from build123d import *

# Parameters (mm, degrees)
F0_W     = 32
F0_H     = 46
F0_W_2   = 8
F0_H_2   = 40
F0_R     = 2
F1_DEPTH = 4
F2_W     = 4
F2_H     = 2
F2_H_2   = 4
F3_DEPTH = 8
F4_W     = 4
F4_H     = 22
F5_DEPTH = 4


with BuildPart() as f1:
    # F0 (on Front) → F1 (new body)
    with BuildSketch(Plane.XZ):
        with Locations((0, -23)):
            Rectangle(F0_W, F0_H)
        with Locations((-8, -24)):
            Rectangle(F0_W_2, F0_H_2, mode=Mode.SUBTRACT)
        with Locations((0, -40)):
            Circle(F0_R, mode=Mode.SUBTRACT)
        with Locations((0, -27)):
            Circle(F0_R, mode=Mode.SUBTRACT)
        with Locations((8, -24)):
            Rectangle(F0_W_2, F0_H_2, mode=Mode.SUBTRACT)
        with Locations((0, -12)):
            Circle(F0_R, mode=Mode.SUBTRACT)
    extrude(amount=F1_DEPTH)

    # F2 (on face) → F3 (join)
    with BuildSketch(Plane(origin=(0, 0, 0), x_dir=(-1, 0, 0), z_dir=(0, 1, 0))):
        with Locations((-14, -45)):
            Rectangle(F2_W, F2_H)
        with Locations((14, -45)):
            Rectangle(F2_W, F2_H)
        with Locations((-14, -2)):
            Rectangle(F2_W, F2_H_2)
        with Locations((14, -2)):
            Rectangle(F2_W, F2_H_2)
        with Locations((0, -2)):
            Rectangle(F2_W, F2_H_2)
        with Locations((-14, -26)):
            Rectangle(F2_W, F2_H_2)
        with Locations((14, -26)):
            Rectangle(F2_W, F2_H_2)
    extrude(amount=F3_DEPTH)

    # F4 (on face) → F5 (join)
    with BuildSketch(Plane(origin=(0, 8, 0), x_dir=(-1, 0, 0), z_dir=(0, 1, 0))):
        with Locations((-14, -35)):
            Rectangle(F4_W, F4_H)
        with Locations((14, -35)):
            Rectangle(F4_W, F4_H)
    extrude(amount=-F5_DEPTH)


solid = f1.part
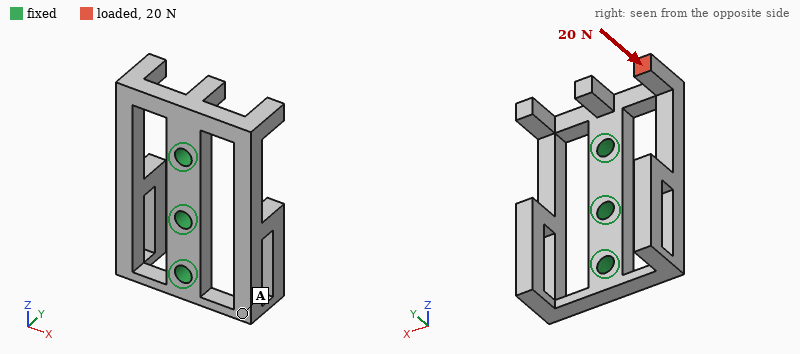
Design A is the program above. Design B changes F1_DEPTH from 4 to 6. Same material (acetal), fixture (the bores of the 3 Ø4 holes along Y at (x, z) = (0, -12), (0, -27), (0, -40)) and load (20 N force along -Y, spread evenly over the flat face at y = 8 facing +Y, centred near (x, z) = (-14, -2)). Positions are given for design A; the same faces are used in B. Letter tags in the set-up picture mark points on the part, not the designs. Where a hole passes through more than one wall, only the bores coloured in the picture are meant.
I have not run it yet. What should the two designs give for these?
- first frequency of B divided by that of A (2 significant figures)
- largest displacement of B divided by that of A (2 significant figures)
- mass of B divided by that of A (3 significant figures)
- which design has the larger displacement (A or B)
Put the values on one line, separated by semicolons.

1.4; 0.39; 1.36; A
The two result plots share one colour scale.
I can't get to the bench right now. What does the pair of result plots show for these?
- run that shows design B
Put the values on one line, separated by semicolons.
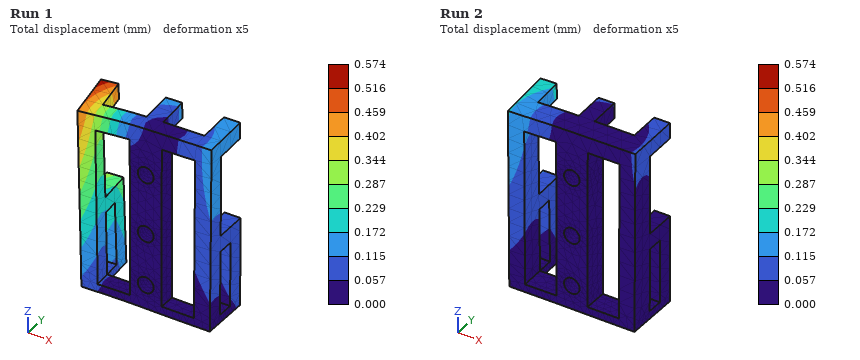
Run 2
